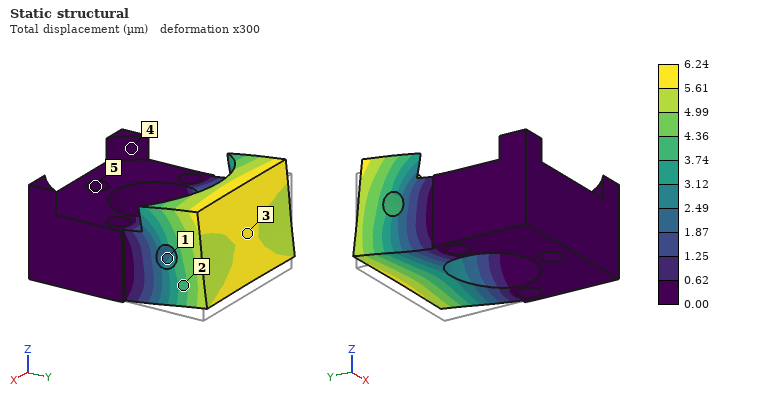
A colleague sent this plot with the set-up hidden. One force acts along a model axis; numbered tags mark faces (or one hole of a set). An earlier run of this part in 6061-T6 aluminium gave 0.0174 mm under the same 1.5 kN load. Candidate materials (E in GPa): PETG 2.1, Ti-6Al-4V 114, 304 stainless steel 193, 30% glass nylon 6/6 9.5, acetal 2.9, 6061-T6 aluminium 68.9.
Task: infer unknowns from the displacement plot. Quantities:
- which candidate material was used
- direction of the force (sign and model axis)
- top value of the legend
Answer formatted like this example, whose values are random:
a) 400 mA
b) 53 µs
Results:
a) 304 stainless steel
b) +Z
c) 6.24 µm
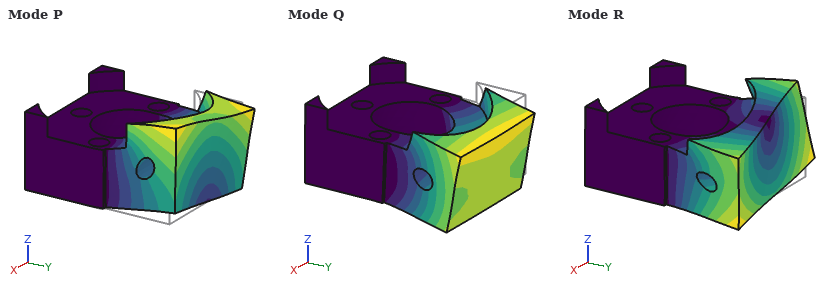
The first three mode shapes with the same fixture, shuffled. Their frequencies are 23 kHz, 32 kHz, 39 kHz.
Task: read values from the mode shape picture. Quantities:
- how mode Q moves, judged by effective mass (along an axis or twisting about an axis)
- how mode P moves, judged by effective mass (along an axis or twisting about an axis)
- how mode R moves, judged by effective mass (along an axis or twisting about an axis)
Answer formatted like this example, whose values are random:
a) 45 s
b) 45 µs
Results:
a) along Z
b) along X
c) along X
